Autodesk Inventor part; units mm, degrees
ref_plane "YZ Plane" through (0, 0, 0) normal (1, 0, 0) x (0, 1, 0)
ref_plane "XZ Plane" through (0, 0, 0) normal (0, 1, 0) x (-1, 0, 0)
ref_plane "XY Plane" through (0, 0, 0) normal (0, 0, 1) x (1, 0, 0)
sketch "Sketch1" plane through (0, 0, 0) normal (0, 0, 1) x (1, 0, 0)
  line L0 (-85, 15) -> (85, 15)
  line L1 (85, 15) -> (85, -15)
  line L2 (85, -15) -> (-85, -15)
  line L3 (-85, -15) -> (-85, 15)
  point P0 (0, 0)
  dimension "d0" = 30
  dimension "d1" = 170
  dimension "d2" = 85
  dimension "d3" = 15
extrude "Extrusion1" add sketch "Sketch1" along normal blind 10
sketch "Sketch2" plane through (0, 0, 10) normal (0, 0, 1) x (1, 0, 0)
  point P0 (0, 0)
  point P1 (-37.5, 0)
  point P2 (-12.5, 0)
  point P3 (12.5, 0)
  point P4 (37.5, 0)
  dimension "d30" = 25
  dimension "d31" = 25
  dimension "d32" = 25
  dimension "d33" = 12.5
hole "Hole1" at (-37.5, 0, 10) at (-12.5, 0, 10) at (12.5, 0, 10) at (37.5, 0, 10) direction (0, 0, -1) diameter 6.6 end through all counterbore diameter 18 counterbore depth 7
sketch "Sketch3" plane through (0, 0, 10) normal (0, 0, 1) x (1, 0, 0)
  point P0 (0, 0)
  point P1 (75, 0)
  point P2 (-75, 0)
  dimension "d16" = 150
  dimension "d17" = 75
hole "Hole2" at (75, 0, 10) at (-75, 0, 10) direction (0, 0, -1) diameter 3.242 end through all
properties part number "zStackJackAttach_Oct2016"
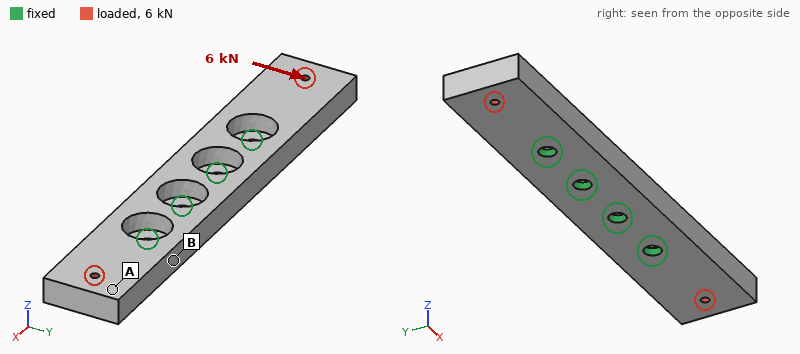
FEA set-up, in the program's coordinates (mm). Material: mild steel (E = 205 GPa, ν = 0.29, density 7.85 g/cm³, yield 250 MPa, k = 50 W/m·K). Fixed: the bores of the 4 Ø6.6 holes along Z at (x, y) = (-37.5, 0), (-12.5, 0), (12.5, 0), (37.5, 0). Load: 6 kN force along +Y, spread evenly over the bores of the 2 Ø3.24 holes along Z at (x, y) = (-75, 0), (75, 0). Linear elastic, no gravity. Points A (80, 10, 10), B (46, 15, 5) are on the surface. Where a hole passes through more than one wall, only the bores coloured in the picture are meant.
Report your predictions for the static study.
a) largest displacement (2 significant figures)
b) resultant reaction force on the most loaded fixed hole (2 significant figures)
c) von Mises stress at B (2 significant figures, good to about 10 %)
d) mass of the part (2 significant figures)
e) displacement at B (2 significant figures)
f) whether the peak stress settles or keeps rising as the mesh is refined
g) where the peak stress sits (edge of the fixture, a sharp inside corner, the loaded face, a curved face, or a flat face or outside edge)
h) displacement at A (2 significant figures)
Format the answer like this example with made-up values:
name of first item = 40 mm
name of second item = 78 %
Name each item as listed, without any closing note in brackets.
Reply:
largest displacement = 59 µm
resultant reaction force on the most loaded fixed hole = 5.2 kN
von Mises stress at B = 64 MPa
mass of the part = 340 g
displacement at B = 20 µm
whether the peak stress settles or keeps rising as the mesh is refined = keeps rising
where the peak stress sits = edge of the fixture
displacement at A = 53 µm
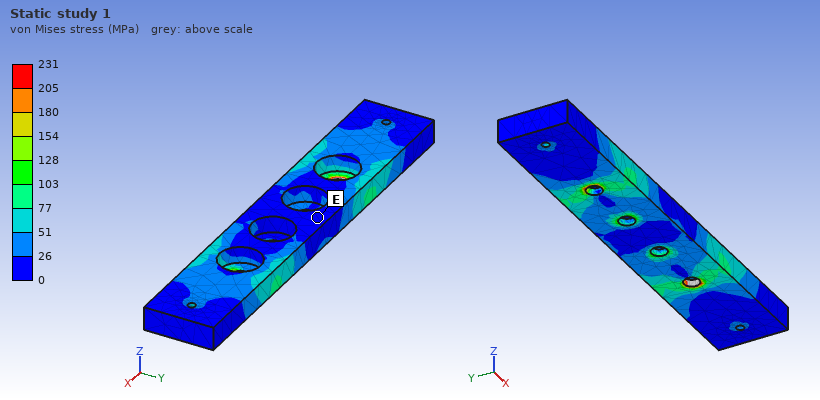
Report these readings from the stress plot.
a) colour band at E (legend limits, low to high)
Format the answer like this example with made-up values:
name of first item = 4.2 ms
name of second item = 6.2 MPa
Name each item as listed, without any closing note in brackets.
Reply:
colour band at E = 0 to 26 MPa
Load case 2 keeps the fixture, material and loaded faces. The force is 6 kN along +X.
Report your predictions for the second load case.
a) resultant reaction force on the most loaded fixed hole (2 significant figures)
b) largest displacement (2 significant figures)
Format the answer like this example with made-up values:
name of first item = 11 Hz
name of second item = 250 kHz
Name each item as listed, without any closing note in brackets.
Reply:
resultant reaction force on the most loaded fixed hole = 1.9 kN
largest displacement = 17 µm
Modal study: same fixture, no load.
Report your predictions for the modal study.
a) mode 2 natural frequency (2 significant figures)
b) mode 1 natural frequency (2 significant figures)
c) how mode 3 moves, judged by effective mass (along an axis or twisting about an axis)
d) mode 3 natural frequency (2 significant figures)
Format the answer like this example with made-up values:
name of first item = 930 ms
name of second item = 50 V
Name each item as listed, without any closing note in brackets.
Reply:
mode 2 natural frequency = 2400 Hz
mode 1 natural frequency = 2400 Hz
how mode 3 moves, judged by effective mass = along Y
mode 3 natural frequency = 4500 Hz
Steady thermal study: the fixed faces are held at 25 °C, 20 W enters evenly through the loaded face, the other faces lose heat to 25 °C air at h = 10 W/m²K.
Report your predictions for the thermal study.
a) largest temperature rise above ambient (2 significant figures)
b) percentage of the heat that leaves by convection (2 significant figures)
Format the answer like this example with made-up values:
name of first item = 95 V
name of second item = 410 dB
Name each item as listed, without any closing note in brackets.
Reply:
largest temperature rise above ambient = 37 K
percentage of the heat that leaves by convection = 11 %
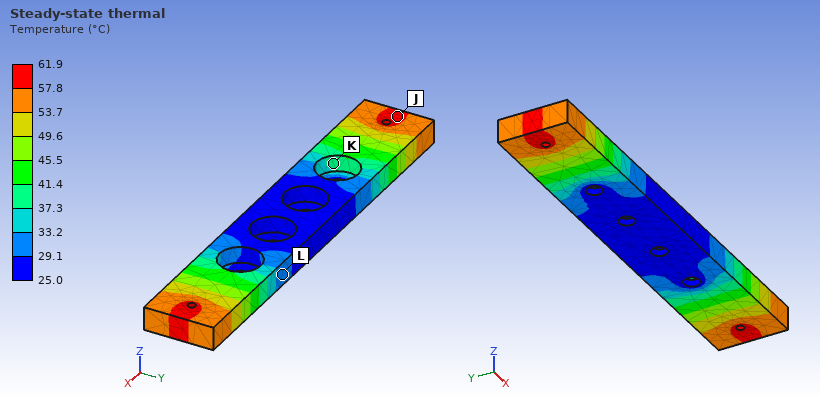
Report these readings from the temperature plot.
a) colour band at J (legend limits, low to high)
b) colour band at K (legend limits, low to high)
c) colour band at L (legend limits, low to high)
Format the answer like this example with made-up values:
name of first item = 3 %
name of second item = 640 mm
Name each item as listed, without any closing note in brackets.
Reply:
colour band at J = 57.8 to 61.9 °C
colour band at K = 37.3 to 41.4 °C
colour band at L = 29.1 to 33.2 °C
